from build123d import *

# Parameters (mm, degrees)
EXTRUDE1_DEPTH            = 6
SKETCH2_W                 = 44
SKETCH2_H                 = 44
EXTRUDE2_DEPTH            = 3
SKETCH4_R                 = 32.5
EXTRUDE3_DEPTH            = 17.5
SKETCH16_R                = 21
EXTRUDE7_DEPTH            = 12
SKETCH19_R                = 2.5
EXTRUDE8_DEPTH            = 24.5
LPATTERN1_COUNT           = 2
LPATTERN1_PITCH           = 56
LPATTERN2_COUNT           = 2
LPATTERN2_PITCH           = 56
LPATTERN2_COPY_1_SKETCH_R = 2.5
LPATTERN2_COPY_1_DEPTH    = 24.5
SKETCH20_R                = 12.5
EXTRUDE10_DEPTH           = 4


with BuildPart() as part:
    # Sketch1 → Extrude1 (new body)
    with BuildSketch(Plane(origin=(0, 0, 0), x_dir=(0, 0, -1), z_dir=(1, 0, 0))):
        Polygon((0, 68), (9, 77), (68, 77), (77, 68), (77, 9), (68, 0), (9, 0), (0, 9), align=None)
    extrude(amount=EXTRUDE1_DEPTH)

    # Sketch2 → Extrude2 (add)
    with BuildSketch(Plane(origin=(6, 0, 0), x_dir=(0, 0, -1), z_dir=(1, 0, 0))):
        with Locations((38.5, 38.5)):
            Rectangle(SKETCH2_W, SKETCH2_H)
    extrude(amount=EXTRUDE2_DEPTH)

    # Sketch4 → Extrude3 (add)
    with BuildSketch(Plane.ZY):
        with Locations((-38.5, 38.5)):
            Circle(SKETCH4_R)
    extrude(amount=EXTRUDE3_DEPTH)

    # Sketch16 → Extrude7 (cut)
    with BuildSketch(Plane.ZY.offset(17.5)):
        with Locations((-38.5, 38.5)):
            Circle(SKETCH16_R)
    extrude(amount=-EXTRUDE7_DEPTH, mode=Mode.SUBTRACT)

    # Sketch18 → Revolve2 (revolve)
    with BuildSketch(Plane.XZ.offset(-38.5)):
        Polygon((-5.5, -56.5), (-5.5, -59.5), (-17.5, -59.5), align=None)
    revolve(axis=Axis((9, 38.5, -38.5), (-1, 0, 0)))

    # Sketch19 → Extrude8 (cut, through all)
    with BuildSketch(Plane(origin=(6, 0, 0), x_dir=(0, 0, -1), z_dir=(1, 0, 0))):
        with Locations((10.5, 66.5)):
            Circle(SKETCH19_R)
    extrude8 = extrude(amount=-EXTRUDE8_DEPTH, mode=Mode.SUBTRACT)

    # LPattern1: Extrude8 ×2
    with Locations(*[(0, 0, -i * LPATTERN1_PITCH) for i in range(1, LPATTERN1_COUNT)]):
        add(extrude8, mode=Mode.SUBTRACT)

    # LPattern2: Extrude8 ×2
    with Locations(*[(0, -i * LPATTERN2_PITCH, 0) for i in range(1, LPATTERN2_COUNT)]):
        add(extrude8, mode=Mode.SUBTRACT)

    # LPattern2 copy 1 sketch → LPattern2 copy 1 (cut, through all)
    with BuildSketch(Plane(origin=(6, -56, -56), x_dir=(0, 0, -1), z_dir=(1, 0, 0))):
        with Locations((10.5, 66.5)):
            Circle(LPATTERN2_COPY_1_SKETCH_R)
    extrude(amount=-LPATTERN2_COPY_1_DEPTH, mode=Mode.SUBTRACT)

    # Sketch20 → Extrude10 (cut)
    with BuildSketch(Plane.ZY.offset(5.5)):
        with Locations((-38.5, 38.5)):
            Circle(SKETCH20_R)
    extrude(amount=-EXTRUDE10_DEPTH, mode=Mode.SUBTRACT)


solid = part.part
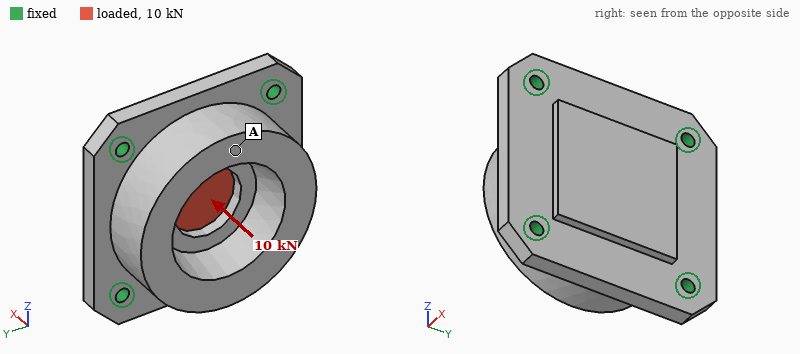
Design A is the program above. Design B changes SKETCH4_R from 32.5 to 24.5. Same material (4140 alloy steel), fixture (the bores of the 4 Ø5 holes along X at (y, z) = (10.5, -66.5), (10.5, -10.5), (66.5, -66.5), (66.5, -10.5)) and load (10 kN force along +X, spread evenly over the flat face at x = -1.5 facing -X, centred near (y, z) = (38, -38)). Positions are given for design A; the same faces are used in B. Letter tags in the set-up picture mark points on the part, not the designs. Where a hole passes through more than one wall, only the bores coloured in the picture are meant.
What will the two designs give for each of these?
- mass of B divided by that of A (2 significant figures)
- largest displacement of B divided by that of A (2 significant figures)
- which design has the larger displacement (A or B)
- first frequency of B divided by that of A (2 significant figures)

0.69
1.8
B
0.84
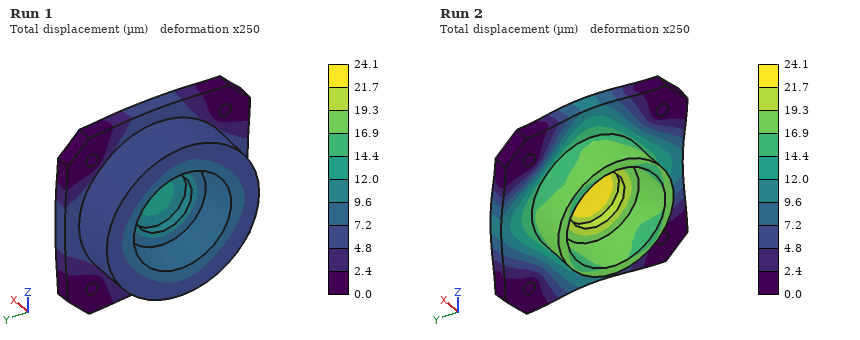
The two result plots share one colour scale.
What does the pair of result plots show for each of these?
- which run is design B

Run 2
